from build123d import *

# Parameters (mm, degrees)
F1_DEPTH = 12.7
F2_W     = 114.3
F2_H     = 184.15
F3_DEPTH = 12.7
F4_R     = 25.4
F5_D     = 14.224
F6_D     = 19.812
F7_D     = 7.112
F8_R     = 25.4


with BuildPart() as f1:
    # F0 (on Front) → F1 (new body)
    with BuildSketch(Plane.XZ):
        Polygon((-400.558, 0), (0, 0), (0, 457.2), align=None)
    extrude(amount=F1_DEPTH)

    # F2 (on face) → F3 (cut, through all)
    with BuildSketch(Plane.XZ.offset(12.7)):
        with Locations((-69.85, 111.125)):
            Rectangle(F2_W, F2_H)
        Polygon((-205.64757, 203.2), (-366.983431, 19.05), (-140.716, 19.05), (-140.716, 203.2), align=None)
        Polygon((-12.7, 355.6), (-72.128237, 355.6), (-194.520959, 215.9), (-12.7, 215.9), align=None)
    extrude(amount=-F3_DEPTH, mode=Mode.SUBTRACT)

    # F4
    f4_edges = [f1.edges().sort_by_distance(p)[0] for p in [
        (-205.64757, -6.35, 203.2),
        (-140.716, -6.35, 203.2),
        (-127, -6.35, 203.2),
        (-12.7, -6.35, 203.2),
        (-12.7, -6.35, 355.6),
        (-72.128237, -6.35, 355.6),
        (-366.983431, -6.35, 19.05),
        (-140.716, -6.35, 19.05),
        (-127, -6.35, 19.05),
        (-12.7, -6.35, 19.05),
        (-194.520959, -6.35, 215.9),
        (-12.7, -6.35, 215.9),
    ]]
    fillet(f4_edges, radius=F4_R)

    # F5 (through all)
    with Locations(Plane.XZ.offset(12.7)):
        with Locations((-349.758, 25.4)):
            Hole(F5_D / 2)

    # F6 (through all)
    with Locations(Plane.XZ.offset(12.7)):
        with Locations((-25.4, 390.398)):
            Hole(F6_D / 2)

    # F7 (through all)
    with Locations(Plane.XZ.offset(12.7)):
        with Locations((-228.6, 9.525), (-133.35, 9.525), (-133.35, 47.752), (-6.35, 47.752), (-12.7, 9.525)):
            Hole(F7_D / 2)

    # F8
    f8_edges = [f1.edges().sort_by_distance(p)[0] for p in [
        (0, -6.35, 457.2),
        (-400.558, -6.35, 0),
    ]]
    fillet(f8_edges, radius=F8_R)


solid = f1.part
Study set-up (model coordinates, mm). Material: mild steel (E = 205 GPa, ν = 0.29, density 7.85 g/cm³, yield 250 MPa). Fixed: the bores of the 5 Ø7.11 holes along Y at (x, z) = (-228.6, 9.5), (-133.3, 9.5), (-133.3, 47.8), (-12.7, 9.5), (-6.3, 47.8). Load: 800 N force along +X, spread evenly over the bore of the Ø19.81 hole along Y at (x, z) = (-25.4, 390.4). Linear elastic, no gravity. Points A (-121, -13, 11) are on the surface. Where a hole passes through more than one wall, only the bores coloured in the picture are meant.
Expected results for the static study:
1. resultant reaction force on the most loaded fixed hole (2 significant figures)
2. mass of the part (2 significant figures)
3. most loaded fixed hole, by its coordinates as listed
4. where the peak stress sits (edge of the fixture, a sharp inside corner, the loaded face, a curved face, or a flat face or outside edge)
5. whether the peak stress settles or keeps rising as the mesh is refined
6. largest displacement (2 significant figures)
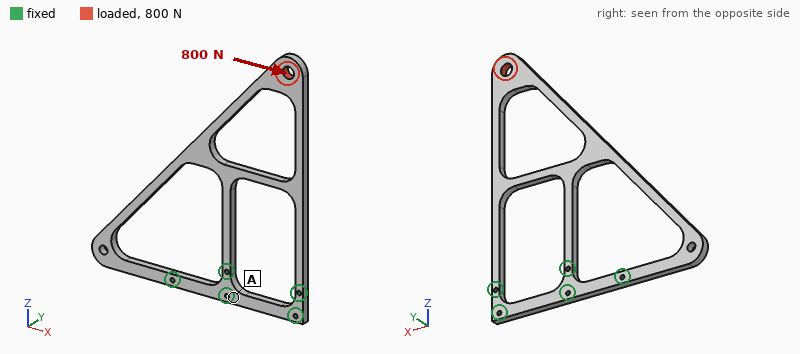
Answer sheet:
1.2 kN
2.7 kg
(-6.3, 47.8)
edge of the fixture
keeps rising
0.31 mm
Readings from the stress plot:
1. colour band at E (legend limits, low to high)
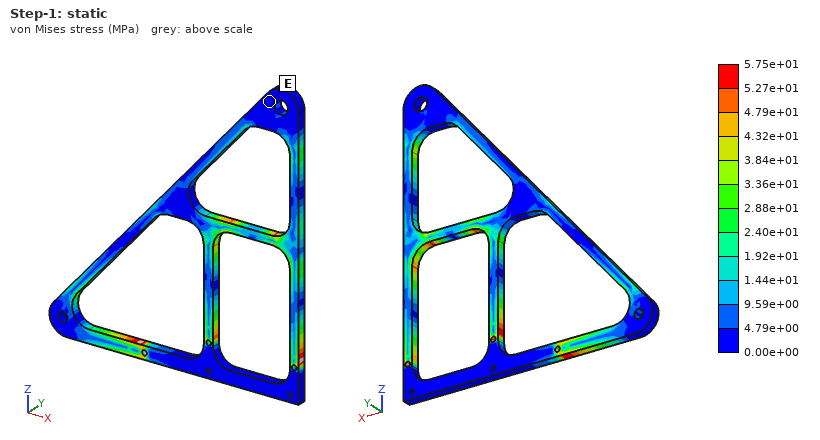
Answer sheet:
0.00e+00 to 4.79e+00 MPa
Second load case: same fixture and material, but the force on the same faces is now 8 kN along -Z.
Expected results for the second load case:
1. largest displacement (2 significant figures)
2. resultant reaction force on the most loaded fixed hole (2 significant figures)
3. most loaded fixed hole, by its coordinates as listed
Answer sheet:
0.19 mm
6.9 kN
(-6.3, 47.8)
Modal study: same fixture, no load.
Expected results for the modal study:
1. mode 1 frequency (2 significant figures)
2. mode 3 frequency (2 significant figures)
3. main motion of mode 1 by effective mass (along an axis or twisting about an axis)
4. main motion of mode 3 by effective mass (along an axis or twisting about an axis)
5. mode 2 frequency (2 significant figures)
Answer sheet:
65 Hz
240 Hz
along Y
along X
210 Hz
